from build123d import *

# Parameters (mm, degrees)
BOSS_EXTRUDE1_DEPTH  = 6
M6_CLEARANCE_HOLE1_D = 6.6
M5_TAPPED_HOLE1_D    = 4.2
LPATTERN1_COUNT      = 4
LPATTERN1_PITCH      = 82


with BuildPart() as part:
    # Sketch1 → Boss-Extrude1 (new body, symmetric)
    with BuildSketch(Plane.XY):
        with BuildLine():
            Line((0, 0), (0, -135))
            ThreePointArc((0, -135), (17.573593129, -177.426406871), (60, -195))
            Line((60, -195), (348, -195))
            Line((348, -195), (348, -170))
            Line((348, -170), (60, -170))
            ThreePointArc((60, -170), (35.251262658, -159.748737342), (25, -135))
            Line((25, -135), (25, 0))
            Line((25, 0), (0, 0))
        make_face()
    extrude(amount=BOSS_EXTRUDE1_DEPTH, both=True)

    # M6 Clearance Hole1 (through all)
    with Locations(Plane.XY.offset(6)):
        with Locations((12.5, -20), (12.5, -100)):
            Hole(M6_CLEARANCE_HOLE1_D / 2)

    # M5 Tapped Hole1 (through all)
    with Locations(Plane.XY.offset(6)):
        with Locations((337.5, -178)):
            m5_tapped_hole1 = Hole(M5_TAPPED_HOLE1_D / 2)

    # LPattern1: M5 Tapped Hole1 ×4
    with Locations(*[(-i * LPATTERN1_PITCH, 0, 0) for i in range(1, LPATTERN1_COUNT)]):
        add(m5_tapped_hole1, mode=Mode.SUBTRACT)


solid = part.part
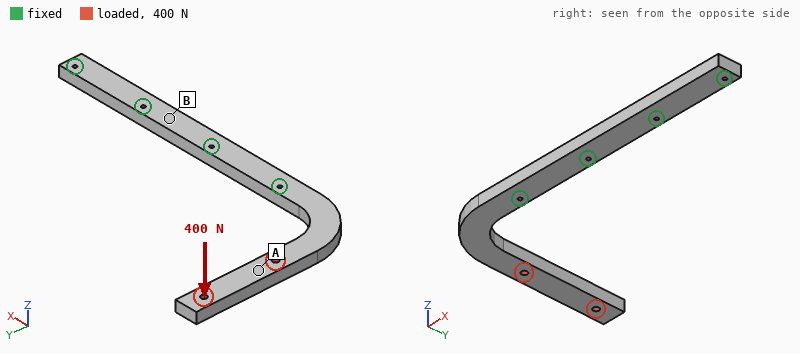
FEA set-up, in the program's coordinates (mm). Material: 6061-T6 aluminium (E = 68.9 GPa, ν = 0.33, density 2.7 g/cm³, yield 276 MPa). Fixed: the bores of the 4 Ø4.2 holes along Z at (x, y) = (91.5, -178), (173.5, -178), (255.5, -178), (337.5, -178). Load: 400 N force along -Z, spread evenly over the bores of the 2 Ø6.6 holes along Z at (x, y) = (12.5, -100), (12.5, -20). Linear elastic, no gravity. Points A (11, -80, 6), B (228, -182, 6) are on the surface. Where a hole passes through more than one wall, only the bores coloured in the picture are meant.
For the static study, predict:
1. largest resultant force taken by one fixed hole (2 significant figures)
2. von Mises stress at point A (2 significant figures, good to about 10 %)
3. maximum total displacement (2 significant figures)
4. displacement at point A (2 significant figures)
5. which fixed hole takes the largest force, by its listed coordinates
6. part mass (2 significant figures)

440 N
20 MPa
4.1 mm
2.1 mm
(91.5, -178)
400 g
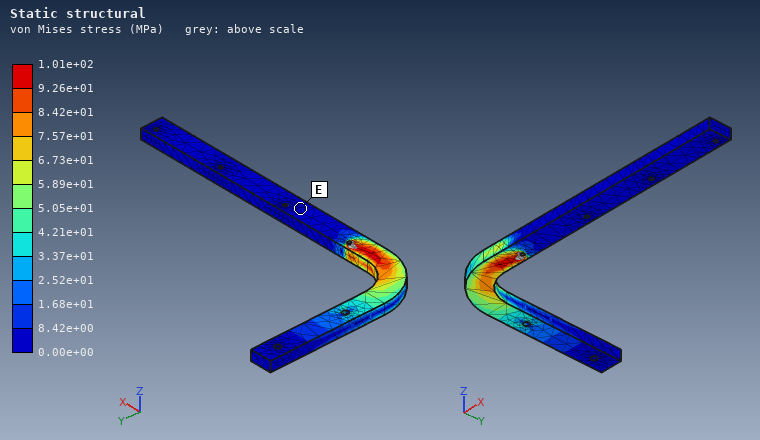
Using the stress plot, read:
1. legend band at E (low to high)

0.00e+00 to 8.42e+00 MPa
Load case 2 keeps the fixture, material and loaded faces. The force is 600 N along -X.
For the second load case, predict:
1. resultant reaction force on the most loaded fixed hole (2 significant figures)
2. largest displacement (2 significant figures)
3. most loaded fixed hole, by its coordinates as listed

2.0 kN
1.6 mm
(91.5, -178)
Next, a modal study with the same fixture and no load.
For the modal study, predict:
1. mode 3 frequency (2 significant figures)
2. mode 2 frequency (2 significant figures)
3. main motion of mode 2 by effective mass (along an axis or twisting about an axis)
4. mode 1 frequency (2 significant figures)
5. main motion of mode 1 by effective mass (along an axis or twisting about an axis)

810 Hz
360 Hz
along X
190 Hz
along Z
